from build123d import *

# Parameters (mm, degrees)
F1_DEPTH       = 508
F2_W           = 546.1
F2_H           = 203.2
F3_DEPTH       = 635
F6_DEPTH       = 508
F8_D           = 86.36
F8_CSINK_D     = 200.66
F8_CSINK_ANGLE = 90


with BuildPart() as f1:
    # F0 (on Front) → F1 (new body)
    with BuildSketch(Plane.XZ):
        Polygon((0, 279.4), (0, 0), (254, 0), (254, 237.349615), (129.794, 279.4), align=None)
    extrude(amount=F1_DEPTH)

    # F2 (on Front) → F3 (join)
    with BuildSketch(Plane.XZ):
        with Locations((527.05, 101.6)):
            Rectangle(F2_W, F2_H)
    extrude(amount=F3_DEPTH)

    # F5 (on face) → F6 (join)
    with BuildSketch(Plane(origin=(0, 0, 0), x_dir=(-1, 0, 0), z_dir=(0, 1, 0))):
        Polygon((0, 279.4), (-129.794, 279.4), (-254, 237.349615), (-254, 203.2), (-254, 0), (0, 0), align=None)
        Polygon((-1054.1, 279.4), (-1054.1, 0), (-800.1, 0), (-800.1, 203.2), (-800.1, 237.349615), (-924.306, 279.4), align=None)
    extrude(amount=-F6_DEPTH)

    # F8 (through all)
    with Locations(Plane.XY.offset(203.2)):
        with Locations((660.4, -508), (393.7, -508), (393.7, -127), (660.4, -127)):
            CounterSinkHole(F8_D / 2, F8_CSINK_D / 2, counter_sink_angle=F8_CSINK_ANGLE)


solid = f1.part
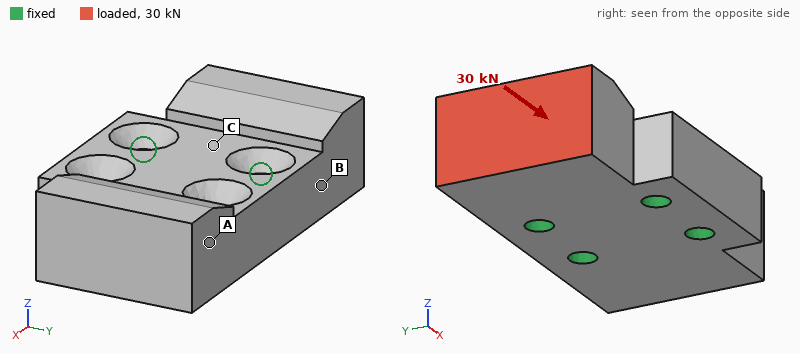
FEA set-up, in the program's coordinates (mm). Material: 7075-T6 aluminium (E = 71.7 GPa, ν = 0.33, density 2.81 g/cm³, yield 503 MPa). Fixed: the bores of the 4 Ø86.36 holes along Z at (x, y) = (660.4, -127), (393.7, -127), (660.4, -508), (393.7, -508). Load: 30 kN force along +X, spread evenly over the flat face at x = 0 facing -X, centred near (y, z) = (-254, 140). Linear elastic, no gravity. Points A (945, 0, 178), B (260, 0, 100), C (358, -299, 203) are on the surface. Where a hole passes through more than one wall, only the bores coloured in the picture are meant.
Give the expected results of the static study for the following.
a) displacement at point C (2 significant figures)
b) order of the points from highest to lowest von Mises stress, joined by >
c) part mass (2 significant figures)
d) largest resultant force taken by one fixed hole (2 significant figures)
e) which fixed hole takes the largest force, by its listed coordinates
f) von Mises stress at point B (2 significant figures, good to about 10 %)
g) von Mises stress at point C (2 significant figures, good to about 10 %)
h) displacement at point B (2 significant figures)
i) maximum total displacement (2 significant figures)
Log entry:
1.4 µm
C > B > A
370 kg
15 kN
(393.7, -127)
0.26 MPa
0.45 MPa
1.3 µm
6.4 µm
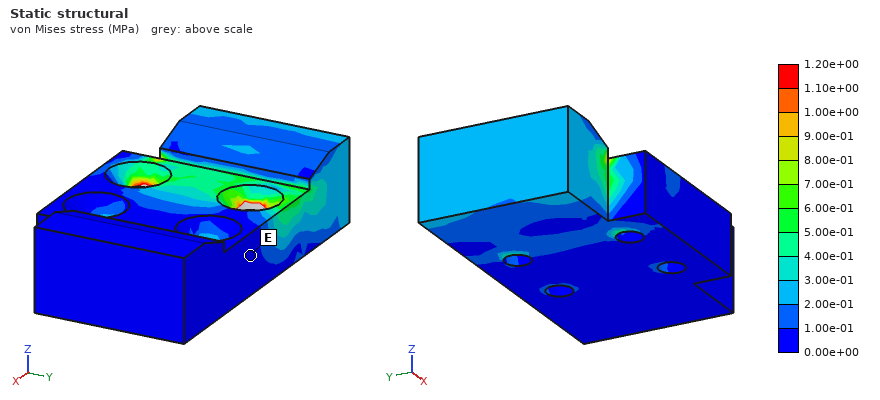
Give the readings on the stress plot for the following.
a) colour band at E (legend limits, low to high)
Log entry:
0.00e+00 to 1.00e-01 MPa
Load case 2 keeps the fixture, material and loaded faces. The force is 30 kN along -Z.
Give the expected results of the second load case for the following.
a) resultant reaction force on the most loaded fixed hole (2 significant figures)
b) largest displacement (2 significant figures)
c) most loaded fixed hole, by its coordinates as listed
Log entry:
27 kN
40 µm
(393.7, -127)
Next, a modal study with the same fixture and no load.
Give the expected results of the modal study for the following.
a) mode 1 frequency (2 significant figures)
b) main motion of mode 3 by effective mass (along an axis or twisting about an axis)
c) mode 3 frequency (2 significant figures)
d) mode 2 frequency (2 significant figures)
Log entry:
650 Hz
twisting about Z
1300 Hz
670 Hz
